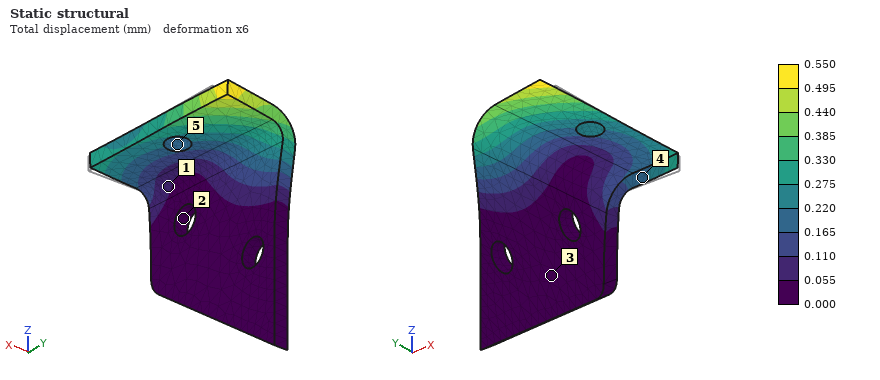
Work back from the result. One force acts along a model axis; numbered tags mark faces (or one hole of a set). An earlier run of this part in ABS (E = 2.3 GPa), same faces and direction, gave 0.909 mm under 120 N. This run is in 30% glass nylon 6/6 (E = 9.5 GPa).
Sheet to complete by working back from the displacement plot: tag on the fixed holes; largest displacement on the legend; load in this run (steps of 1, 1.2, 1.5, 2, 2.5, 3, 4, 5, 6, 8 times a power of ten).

2
0.550 mm
300 N
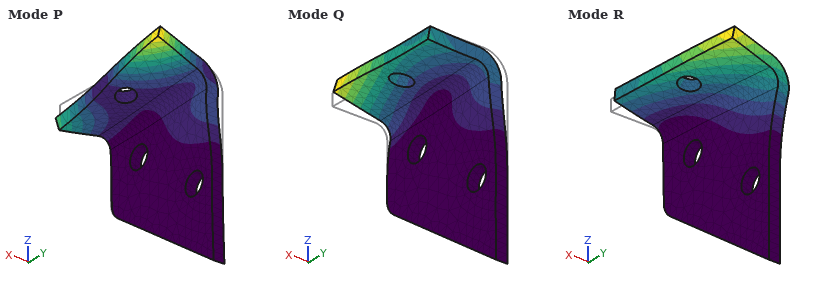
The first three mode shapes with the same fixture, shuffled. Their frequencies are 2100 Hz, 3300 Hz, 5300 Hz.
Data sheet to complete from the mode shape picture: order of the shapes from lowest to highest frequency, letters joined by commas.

R, Q, P
